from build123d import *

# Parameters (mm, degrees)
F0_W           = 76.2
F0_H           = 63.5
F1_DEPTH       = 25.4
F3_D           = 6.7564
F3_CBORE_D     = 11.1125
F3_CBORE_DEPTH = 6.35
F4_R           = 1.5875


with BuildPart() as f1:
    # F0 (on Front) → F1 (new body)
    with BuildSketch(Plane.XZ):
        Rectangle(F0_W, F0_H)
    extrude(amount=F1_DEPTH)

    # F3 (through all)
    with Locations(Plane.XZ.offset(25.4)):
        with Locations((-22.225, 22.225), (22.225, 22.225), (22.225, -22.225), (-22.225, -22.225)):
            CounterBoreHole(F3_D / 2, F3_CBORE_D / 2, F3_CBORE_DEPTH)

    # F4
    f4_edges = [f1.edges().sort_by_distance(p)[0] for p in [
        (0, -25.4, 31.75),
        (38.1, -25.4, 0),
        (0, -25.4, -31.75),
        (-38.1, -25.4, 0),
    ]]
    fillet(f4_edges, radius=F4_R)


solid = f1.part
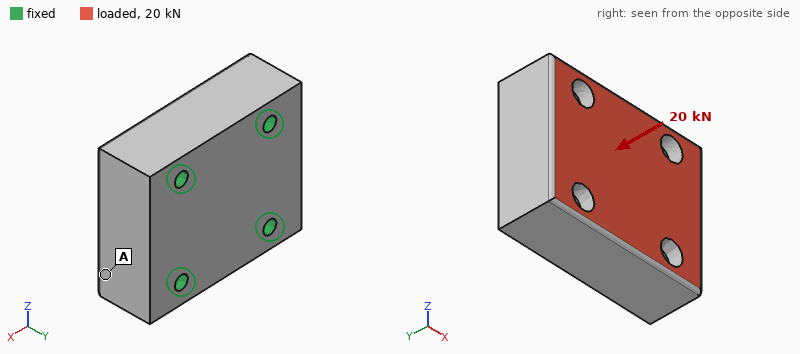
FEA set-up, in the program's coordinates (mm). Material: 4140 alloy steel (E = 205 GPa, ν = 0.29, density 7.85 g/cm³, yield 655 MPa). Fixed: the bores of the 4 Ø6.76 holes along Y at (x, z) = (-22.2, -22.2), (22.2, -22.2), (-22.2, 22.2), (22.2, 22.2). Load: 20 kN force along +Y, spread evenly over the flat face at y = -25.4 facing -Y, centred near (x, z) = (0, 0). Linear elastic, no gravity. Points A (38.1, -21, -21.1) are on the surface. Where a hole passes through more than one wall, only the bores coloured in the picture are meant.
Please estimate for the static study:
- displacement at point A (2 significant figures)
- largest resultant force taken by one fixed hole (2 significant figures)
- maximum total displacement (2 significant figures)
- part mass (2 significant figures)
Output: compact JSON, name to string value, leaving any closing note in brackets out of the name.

{"displacement at point A": "0.88 µm", "largest resultant force taken by one fixed hole": "5.1 kN", "maximum total displacement": "1.8 µm", "part mass": "920 g"}
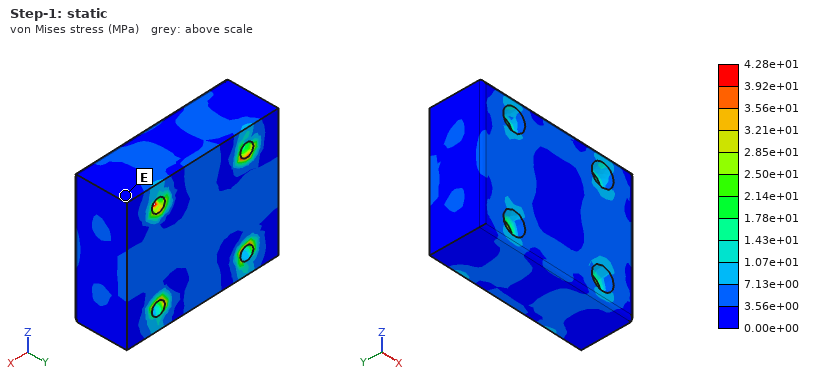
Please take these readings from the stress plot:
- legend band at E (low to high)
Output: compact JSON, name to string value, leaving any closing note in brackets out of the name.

{"legend band at E": "0.00e+00 to 3.56e+00 MPa"}
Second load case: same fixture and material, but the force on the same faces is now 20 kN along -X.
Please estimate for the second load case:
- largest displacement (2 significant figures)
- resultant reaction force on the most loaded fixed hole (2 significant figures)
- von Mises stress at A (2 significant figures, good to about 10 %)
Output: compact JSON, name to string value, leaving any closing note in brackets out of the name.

{"largest displacement": "3.2 µm", "resultant reaction force on the most loaded fixed hole": "5.6 kN", "von Mises stress at A": "6.8 MPa"}
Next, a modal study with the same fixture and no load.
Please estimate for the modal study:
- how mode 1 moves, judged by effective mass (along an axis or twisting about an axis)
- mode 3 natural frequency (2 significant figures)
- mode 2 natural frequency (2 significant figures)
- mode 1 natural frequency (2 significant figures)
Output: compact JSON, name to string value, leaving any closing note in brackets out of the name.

{"how mode 1 moves, judged by effective mass": "along Y", "mode 3 natural frequency": "25 kHz", "mode 2 natural frequency": "23 kHz", "mode 1 natural frequency": "22 kHz"}
